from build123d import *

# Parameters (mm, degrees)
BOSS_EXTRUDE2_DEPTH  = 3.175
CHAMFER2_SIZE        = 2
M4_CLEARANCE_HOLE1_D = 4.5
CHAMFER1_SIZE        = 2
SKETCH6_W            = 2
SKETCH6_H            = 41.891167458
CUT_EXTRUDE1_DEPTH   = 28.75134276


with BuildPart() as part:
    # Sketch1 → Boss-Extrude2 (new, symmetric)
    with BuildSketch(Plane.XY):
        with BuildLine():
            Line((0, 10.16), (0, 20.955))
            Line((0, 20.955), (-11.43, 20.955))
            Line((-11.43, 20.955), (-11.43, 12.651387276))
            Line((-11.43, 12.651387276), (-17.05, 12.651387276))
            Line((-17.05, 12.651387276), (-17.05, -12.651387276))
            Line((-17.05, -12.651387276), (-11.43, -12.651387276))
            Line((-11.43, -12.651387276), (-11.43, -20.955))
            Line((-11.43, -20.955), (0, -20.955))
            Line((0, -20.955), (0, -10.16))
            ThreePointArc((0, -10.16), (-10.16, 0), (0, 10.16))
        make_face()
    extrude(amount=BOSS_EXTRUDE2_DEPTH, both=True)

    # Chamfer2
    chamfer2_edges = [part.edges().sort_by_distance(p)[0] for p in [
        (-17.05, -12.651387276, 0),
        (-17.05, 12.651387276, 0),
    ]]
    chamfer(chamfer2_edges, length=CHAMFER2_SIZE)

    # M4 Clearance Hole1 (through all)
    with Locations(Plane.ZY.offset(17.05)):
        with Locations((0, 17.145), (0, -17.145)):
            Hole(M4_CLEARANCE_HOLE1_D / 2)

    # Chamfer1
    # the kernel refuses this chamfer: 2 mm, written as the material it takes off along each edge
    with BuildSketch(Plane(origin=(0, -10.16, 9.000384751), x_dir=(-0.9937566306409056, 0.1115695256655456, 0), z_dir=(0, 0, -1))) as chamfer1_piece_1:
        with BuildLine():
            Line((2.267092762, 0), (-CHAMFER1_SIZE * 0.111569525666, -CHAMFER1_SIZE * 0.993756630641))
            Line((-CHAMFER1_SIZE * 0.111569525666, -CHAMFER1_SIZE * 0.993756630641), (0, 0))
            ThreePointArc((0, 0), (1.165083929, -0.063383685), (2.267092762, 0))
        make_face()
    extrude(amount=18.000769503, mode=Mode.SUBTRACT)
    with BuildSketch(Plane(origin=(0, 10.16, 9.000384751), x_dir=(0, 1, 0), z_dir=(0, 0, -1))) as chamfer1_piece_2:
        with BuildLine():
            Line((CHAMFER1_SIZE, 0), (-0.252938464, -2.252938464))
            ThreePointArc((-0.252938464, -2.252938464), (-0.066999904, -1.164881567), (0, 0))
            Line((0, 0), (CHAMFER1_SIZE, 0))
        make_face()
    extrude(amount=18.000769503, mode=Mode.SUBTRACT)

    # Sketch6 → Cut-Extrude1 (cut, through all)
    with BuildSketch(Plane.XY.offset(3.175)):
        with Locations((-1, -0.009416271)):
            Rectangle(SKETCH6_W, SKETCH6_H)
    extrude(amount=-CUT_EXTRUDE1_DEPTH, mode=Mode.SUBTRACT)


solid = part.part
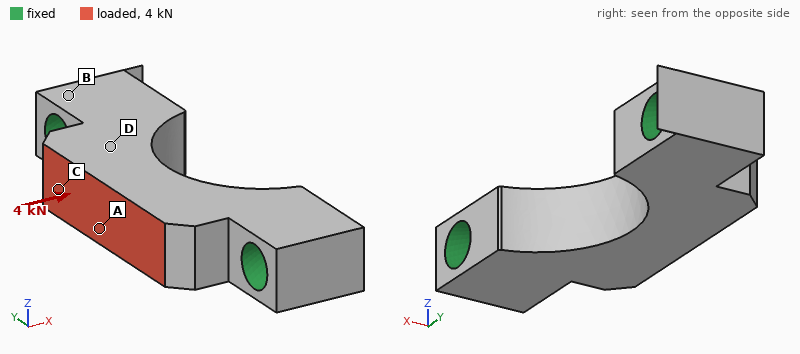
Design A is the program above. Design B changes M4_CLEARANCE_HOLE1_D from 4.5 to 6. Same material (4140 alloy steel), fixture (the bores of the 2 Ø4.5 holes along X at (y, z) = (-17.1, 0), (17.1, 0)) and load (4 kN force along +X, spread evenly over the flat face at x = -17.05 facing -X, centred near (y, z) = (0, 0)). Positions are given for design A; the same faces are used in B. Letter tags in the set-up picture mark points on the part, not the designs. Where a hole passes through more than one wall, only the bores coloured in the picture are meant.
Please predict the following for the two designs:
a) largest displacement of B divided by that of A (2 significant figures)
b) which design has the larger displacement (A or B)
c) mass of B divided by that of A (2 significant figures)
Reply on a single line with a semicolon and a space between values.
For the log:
0.91; A; 0.90
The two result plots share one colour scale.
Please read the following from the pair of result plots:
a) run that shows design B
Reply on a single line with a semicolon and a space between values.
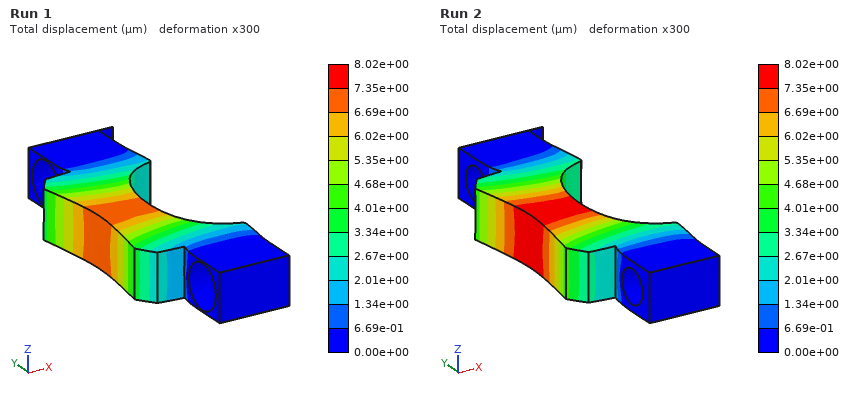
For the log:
Run 1
